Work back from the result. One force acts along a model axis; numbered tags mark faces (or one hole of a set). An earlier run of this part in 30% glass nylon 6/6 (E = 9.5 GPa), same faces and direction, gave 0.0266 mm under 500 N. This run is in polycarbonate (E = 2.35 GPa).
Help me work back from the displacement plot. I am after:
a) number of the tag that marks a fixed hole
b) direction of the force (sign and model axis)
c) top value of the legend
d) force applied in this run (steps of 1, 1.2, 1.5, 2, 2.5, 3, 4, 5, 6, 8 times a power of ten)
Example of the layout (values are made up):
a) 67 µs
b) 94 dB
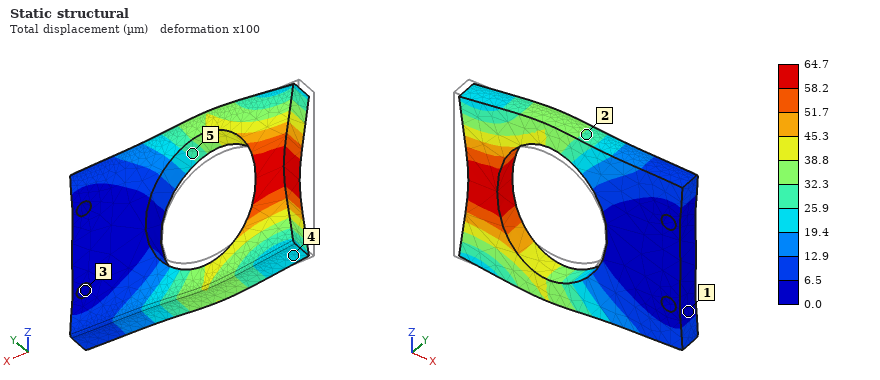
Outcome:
a) 3
b) +X
c) 64.7 µm
d) 300 N
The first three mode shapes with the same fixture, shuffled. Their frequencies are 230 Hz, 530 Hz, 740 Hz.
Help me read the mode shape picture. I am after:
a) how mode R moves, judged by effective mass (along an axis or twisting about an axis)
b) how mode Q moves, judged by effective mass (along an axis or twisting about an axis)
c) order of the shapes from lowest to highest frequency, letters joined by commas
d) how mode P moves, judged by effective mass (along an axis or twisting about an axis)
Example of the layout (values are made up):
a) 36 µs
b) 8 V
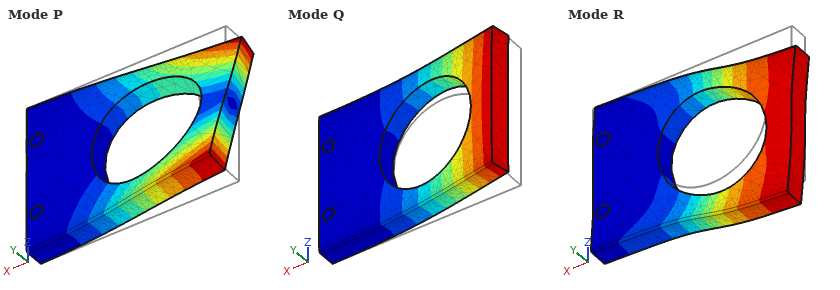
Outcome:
a) along Z
b) along Y
c) Q, P, R
d) twisting about X
